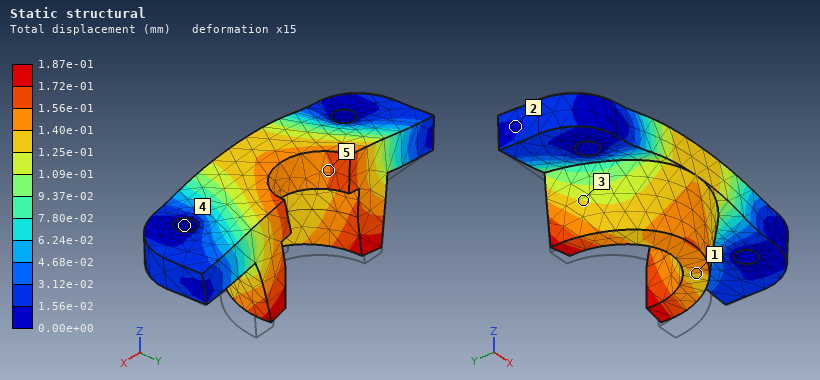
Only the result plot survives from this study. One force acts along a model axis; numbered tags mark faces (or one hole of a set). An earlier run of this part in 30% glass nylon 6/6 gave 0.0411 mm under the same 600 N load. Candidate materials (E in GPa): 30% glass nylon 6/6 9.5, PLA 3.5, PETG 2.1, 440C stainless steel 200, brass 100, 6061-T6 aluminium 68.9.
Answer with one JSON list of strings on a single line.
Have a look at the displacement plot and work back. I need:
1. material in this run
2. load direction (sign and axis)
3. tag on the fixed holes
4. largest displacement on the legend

["PETG", "+Z", "4", "1.87e-01 mm"]
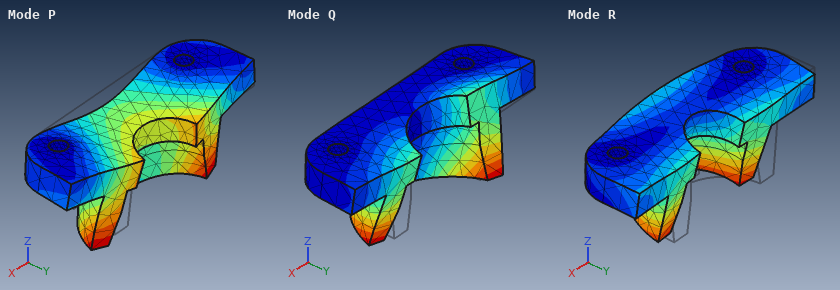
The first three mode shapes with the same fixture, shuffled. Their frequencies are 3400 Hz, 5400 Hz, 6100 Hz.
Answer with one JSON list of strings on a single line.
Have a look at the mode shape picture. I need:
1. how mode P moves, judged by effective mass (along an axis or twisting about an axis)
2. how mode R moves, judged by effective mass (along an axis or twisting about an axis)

["along Z", "along Y"]
